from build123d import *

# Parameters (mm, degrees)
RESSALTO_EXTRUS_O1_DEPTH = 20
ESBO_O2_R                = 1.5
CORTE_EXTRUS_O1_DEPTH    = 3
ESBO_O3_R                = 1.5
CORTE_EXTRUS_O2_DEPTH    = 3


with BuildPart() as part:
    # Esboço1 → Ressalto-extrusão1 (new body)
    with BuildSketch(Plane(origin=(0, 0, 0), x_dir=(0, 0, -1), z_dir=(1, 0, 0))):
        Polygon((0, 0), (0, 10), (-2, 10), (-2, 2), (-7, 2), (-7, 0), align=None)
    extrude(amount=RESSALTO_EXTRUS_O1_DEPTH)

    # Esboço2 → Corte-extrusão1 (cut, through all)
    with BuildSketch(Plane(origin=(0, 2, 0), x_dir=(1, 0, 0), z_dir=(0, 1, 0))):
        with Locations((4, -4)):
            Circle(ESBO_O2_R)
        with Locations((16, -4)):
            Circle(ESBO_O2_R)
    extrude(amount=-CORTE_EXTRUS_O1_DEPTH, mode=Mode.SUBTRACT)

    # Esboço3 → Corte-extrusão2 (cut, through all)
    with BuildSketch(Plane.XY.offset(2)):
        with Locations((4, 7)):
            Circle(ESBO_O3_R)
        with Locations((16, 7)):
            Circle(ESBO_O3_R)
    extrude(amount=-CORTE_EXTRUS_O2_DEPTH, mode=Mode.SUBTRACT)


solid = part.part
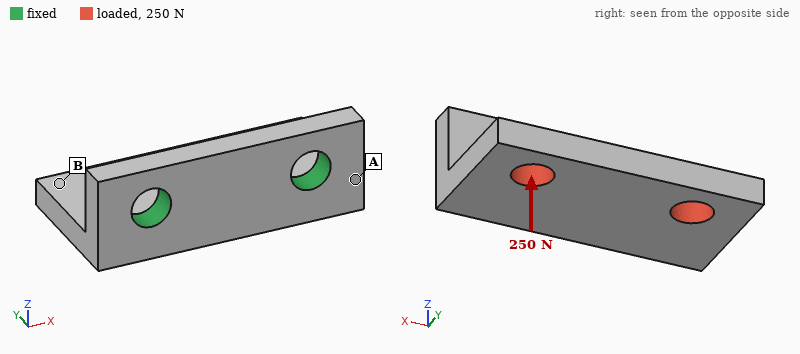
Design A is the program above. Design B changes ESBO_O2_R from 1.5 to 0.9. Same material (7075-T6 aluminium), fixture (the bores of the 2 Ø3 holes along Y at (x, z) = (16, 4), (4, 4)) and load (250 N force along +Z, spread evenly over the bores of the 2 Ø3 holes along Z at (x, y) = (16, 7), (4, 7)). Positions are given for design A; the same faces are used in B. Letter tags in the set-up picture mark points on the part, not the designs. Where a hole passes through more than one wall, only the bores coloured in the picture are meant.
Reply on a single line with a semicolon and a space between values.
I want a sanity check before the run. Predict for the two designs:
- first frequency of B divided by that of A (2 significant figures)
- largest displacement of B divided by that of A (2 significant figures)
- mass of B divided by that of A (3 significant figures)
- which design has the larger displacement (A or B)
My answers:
0.88; 1.2; 1.03; B
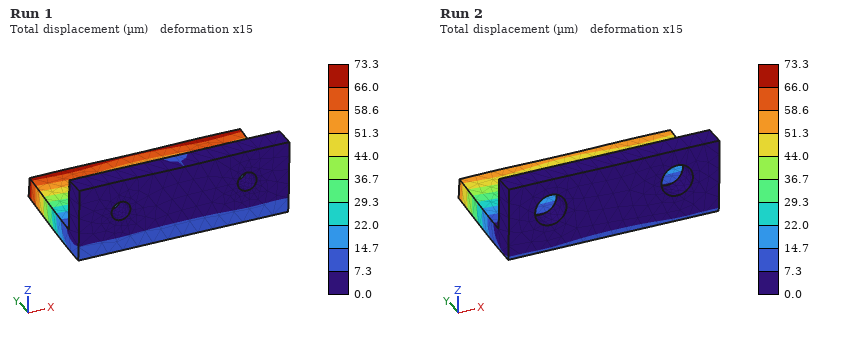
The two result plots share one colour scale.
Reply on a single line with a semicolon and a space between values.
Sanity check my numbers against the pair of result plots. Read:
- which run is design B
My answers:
Run 1
